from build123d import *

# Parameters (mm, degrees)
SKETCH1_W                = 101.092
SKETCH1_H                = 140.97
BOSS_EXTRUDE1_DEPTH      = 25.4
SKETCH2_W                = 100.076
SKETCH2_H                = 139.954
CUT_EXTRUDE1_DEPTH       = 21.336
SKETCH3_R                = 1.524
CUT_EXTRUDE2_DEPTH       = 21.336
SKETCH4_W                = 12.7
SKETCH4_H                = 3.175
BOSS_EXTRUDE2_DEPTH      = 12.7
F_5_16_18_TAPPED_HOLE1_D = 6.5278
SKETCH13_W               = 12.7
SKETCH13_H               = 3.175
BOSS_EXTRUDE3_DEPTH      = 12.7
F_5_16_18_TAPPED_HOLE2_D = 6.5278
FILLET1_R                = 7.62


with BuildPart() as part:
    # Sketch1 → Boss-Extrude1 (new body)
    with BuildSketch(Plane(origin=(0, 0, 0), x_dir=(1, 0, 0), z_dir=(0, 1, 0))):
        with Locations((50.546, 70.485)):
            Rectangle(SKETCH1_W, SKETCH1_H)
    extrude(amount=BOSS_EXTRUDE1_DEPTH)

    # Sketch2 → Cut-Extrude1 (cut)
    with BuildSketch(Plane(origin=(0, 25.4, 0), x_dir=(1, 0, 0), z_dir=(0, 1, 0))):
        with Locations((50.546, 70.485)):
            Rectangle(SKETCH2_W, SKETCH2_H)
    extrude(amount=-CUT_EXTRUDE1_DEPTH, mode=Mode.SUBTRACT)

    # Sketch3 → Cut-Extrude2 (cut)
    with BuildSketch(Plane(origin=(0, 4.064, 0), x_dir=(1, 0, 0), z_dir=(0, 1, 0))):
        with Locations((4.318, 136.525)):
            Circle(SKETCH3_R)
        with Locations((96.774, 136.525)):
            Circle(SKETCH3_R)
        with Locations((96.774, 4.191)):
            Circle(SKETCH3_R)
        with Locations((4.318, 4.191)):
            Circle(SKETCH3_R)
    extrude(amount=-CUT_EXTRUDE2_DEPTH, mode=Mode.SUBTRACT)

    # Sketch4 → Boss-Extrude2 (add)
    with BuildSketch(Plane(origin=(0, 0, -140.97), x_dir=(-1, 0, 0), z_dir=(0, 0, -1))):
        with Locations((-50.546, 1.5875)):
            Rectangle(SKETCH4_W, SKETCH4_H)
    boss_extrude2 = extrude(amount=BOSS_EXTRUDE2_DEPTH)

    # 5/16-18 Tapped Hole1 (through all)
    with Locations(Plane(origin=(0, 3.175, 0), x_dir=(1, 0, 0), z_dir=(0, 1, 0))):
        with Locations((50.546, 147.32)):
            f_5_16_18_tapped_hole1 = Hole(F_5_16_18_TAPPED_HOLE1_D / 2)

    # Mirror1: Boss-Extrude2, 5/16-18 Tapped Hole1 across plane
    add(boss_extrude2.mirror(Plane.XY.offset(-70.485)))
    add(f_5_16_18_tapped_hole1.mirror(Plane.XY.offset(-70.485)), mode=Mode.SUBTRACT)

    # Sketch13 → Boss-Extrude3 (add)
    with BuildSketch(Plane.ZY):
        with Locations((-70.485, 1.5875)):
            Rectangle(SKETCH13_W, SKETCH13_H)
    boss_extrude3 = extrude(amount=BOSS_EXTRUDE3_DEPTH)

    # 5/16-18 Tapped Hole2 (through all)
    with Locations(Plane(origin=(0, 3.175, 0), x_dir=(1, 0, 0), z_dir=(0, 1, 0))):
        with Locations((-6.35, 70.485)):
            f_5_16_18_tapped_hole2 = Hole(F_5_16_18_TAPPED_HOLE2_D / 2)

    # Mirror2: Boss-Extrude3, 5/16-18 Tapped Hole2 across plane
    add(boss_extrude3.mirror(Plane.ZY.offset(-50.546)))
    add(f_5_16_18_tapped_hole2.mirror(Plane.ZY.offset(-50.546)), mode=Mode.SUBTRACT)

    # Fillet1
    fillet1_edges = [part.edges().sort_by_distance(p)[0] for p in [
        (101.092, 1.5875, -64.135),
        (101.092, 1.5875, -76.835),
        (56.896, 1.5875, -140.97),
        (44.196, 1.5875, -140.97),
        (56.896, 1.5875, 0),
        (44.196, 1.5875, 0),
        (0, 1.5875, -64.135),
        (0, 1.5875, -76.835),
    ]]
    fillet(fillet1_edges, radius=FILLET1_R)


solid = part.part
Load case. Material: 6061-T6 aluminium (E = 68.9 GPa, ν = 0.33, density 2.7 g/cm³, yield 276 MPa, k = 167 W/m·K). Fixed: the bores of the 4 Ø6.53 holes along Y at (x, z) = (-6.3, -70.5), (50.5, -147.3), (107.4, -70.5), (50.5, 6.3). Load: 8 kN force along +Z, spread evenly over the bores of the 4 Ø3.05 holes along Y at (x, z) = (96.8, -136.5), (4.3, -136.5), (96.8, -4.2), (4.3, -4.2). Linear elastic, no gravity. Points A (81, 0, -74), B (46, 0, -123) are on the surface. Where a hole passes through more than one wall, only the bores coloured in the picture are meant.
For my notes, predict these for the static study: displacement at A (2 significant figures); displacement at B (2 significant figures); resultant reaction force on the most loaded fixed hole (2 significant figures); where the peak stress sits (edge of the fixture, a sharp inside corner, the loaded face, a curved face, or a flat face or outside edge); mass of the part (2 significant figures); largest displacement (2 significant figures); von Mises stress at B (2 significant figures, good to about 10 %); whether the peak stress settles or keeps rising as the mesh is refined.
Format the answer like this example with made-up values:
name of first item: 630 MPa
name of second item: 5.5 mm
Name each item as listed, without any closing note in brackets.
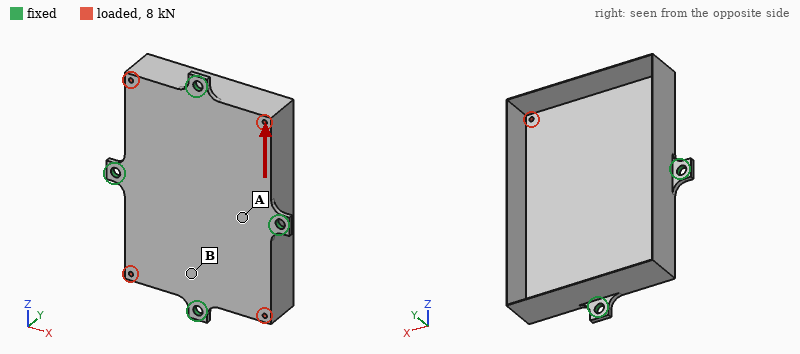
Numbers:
displacement at A: 14 µm
displacement at B: 8.5 µm
resultant reaction force on the most loaded fixed hole: 2.2 kN
where the peak stress sits: edge of the fixture
mass of the part: 180 g
largest displacement: 42 µm
von Mises stress at B: 16 MPa
whether the peak stress settles or keeps rising as the mesh is refined: keeps rising
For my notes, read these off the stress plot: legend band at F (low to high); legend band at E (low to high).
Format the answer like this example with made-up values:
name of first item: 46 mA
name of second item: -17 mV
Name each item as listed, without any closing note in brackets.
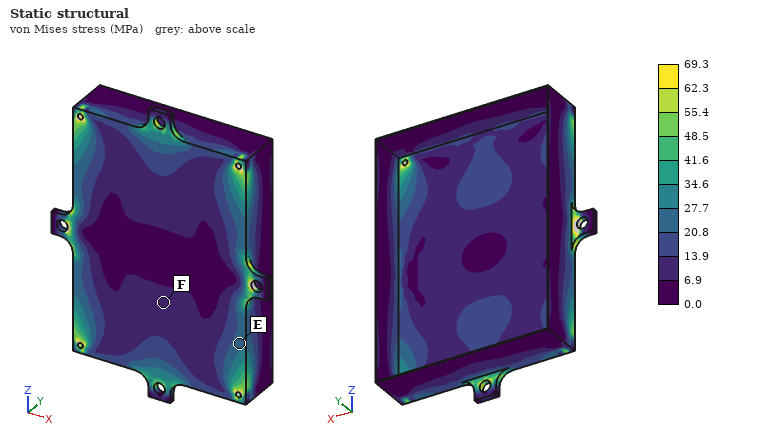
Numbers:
legend band at F: 6.9 to 13.9 MPa
legend band at E: 20.8 to 27.7 MPa
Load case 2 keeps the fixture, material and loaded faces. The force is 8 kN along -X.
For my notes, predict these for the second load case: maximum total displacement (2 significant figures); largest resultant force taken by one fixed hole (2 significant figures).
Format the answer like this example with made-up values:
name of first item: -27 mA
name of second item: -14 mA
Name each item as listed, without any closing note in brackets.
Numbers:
maximum total displacement: 43 µm
largest resultant force taken by one fixed hole: 2.4 kN
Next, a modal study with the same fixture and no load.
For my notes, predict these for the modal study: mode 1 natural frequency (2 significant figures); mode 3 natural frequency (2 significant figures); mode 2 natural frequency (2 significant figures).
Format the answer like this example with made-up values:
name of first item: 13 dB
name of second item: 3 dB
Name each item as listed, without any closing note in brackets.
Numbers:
mode 1 natural frequency: 1200 Hz
mode 3 natural frequency: 1200 Hz
mode 2 natural frequency: 1200 Hz
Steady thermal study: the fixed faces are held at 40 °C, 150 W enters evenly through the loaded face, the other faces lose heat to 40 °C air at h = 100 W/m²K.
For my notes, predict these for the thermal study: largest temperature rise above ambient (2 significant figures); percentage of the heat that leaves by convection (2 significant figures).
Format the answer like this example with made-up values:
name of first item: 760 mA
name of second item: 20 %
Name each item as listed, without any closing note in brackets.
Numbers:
largest temperature rise above ambient: 72 K
percentage of the heat that leaves by convection: 68 %
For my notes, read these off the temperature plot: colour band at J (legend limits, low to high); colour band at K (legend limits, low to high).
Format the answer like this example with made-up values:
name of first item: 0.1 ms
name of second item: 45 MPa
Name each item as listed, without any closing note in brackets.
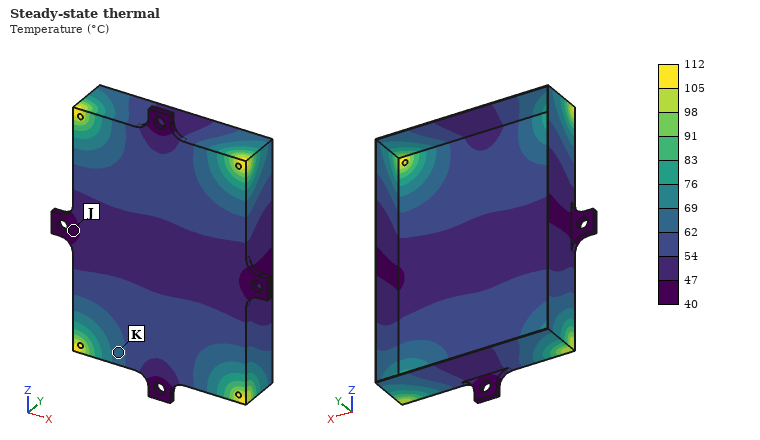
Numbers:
colour band at J: 40 to 47 °C
colour band at K: 62 to 69 °C
